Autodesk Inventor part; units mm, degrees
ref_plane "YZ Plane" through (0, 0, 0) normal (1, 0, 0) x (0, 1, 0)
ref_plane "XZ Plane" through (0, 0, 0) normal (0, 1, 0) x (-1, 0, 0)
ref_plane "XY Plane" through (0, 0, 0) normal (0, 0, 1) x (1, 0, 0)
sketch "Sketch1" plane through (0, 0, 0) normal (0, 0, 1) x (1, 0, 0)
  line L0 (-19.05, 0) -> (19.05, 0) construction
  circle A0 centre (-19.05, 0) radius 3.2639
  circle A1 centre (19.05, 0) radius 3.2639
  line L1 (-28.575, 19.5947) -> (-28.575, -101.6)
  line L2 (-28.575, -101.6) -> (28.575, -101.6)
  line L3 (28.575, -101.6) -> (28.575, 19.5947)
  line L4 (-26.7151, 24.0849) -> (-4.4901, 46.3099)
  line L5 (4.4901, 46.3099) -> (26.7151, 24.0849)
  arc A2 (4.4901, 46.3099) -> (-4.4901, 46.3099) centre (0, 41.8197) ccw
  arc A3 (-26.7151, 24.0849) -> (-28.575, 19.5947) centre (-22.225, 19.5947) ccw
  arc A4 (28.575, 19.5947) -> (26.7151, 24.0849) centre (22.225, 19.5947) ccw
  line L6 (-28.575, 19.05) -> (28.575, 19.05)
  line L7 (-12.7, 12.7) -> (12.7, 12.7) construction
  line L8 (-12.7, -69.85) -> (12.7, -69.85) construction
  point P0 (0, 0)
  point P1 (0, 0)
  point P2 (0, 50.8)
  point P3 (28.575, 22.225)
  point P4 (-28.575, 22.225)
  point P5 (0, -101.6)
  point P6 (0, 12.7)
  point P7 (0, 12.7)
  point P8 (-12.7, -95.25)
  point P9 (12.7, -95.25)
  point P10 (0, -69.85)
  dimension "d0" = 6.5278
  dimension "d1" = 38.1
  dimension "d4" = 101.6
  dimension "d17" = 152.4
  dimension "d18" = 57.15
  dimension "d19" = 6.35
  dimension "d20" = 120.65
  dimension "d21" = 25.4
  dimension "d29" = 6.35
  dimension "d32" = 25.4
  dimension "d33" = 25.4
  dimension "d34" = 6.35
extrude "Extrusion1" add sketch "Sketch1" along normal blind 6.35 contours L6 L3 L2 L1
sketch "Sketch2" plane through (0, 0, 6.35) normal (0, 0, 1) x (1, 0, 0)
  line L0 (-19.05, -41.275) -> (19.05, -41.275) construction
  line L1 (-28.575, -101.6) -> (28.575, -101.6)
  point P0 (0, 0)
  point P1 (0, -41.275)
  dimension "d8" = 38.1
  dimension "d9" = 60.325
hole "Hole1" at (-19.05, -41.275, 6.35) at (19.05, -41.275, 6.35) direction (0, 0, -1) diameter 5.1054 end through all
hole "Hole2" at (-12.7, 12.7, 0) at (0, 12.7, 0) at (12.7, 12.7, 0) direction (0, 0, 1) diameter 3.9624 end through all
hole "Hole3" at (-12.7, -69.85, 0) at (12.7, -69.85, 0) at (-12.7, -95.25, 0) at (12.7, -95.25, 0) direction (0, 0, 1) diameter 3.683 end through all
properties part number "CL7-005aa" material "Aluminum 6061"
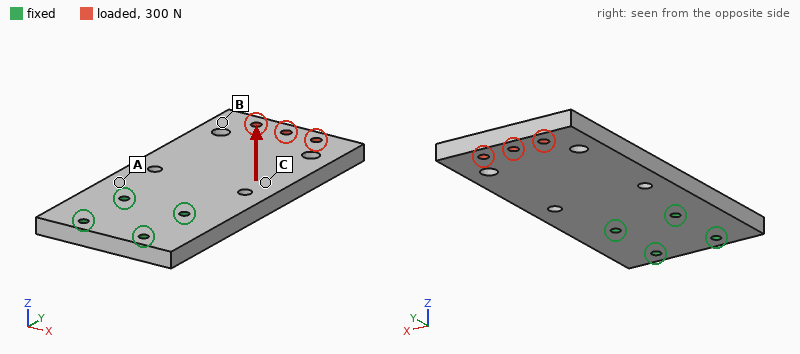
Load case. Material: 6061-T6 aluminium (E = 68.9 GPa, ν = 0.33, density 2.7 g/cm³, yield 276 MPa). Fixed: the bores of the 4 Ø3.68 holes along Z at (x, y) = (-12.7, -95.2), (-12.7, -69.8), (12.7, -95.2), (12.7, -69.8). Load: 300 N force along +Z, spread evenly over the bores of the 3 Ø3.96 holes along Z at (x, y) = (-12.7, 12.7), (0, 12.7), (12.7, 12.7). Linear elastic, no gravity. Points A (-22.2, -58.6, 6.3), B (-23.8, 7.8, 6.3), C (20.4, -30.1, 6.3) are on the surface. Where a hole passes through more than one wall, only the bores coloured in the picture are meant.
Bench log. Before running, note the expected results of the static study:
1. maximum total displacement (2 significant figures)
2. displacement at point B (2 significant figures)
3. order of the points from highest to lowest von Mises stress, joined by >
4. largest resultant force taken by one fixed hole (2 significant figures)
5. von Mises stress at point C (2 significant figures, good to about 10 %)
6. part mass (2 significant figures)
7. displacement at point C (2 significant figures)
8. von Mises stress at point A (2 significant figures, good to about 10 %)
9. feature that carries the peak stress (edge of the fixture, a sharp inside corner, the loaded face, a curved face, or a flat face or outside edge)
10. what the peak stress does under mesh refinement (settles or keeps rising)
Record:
0.80 mm
0.64 mm
A > C > B
350 N
32 MPa
120 g
0.21 mm
52 MPa
edge of the fixture
keeps rising
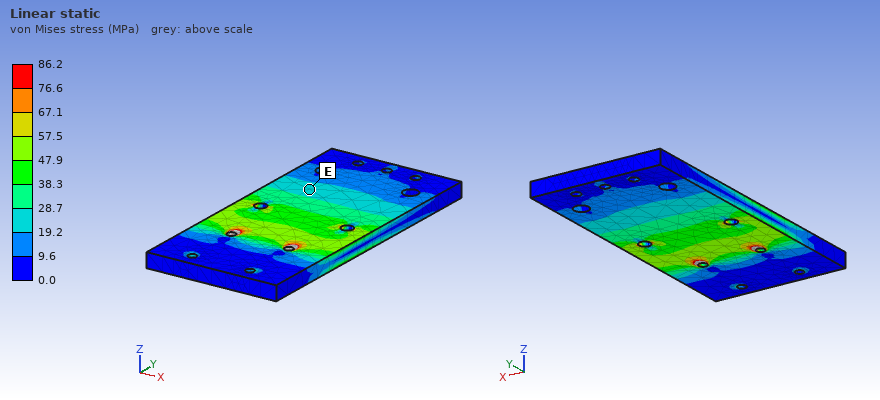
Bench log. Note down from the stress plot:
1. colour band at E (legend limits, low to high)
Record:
19.2 to 28.7 MPa
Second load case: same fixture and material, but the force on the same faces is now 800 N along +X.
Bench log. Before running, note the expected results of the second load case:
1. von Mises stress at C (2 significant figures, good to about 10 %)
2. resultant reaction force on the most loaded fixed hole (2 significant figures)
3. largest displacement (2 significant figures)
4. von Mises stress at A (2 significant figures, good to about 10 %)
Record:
7.1 MPa
1.6 kN
49 µm
11 MPa
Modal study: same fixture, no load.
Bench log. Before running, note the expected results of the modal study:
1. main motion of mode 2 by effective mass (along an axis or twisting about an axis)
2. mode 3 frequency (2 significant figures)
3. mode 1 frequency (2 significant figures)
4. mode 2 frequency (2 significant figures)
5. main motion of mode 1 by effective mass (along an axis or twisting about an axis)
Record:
twisting about Y
3900 Hz
650 Hz
2100 Hz
along Z
